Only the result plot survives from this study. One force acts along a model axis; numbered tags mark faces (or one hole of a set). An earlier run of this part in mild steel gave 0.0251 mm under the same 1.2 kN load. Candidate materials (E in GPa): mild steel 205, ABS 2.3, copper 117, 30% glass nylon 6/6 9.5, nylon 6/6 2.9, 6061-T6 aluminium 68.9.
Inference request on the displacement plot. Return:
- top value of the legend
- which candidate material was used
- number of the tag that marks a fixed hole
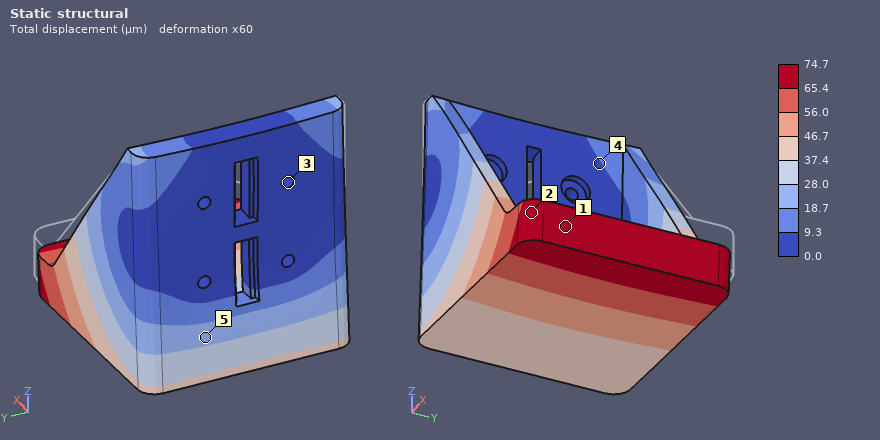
74.7 µm
6061-T6 aluminium
3
